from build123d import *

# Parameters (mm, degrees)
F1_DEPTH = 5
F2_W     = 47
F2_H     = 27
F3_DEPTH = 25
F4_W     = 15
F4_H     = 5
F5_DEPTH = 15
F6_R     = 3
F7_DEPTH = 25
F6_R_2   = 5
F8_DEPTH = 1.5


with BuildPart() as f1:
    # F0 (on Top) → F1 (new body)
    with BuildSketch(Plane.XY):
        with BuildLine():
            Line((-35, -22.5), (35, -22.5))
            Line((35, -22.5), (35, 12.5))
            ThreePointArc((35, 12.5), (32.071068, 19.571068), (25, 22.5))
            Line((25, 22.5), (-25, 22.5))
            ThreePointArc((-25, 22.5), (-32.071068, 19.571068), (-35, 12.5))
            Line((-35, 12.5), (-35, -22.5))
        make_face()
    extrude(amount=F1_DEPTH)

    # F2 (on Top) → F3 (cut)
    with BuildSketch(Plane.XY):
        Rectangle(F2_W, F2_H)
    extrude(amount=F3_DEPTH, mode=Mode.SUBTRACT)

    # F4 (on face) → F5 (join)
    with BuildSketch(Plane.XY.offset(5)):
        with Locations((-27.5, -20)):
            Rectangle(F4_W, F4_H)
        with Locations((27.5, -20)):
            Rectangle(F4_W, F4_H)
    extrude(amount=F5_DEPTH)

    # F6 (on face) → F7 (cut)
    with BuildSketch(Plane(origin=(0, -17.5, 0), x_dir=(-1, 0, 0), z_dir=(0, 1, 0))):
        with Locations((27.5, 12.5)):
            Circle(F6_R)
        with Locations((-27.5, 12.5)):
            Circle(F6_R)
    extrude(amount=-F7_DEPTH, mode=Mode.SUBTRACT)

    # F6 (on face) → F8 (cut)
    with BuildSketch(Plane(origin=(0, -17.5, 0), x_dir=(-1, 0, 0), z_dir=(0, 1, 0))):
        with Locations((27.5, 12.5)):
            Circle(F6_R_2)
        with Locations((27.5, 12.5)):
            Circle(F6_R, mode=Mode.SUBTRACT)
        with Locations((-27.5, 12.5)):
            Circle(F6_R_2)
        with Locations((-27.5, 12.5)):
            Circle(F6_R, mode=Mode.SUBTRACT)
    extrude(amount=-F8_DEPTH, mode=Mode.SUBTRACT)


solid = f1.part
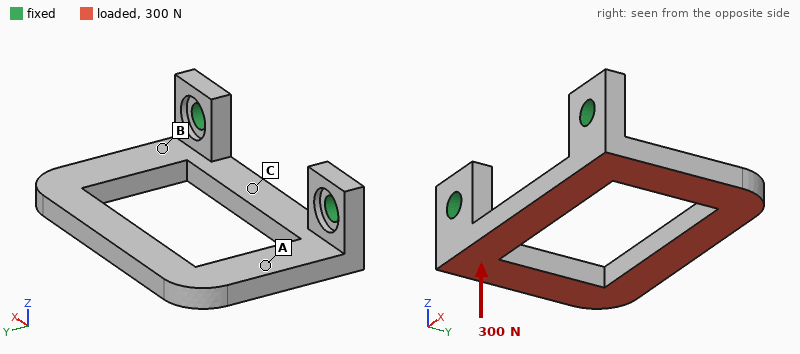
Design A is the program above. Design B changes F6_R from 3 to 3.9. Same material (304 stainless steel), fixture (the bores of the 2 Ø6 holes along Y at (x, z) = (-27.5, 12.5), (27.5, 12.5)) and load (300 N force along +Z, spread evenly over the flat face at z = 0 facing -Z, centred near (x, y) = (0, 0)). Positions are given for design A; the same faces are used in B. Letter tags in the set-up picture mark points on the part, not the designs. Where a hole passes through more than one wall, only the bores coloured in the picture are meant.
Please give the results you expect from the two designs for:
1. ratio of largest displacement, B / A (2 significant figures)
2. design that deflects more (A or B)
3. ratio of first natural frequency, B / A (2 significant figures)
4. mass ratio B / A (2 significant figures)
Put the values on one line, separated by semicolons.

0.92; A; 1.0; 0.99
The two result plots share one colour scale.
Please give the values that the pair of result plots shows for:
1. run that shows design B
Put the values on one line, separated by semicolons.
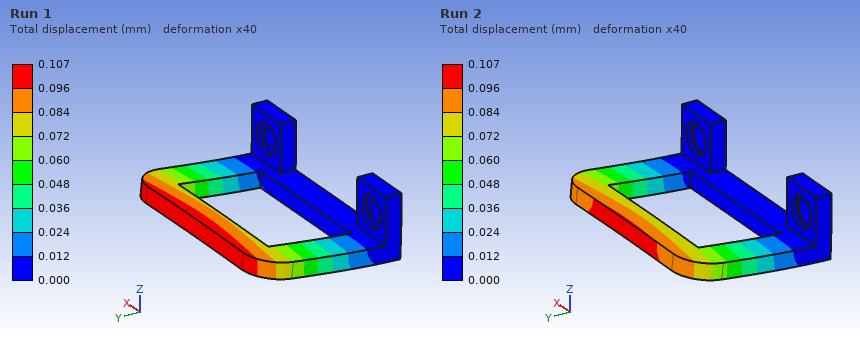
Run 2
